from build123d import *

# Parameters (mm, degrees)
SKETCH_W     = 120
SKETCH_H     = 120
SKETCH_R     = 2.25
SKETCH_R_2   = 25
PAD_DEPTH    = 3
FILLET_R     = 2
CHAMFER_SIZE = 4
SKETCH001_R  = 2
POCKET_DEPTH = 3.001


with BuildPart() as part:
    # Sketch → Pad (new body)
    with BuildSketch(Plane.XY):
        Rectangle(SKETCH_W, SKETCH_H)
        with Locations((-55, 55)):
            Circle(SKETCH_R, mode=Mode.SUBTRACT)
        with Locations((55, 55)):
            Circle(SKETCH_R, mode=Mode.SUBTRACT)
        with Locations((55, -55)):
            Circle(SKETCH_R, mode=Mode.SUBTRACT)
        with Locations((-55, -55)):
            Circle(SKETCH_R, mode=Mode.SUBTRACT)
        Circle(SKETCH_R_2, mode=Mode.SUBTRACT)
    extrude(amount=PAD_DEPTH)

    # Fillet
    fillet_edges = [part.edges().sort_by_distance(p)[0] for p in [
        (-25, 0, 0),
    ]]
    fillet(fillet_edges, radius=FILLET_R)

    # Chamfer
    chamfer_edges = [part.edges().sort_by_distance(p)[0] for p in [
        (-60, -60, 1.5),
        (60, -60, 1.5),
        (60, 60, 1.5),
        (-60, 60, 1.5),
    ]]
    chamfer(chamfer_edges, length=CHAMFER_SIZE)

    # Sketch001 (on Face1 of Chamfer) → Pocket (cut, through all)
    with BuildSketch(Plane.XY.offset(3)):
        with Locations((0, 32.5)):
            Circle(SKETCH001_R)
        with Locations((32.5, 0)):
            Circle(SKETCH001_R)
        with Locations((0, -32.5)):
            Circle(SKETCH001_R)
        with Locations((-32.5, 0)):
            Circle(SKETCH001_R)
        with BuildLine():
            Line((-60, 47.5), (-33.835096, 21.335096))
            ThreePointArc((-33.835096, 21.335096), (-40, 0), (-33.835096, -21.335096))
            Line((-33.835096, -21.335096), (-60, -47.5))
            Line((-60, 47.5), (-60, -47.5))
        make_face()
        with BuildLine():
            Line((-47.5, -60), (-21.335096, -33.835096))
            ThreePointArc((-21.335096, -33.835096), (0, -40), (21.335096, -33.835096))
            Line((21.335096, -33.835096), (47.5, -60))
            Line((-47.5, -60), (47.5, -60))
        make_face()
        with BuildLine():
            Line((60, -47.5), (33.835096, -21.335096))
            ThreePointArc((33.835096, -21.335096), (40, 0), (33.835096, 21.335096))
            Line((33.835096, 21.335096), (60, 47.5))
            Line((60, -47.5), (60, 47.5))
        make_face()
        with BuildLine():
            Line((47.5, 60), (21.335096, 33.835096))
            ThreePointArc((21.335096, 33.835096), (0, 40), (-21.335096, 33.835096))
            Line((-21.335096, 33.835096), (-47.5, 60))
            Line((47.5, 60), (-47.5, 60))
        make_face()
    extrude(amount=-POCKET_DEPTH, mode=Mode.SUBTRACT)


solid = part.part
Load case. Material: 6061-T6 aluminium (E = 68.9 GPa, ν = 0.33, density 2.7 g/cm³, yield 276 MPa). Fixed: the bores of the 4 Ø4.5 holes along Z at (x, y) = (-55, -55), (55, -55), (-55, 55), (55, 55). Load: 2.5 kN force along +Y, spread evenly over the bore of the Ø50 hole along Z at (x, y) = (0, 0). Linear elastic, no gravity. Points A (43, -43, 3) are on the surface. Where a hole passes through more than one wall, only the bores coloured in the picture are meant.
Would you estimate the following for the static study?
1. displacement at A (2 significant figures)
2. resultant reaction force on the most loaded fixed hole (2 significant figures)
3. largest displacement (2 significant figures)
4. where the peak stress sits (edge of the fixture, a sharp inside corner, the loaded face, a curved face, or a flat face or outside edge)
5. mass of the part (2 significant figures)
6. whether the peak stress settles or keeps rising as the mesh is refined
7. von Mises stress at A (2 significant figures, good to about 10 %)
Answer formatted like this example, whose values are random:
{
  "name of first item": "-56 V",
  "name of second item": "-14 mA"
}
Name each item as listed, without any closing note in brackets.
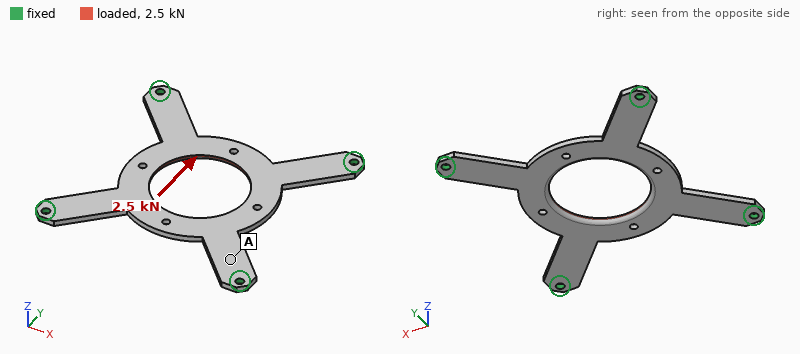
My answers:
{
  "displacement at A": "13 µm",
  "resultant reaction force on the most loaded fixed hole": "830 N",
  "largest displacement": "66 µm",
  "where the peak stress sits": "edge of the fixture",
  "mass of the part": "47 g",
  "whether the peak stress settles or keeps rising as the mesh is refined": "keeps rising",
  "von Mises stress at A": "16 MPa"
}
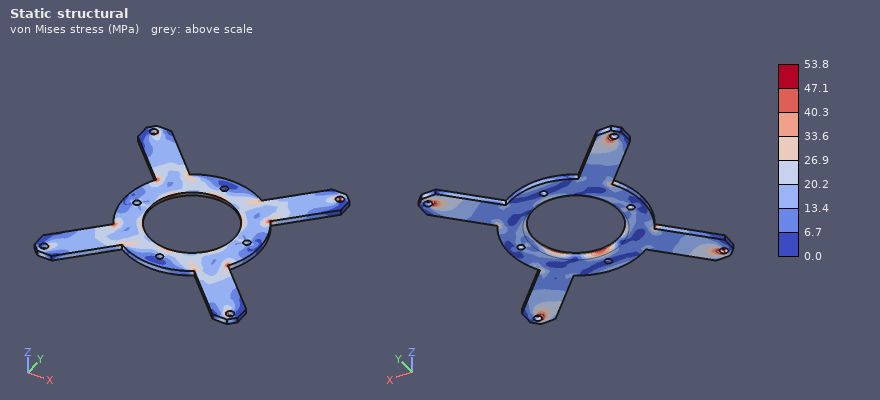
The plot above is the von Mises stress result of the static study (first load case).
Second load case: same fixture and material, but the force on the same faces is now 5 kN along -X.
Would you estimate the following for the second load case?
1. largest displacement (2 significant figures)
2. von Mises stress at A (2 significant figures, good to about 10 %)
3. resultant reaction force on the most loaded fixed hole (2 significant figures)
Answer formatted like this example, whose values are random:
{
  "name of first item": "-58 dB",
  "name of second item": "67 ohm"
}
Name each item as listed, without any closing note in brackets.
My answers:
{
  "largest displacement": "0.13 mm",
  "von Mises stress at A": "33 MPa",
  "resultant reaction force on the most loaded fixed hole": "1.7 kN"
}
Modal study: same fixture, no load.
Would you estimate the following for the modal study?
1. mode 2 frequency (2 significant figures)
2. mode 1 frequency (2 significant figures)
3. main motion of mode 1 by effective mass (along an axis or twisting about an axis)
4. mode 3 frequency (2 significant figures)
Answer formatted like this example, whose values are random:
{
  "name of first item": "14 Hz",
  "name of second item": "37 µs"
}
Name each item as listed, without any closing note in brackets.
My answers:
{
  "mode 2 frequency": "1500 Hz",
  "mode 1 frequency": "800 Hz",
  "main motion of mode 1 by effective mass": "along Z",
  "mode 3 frequency": "1500 Hz"
}
